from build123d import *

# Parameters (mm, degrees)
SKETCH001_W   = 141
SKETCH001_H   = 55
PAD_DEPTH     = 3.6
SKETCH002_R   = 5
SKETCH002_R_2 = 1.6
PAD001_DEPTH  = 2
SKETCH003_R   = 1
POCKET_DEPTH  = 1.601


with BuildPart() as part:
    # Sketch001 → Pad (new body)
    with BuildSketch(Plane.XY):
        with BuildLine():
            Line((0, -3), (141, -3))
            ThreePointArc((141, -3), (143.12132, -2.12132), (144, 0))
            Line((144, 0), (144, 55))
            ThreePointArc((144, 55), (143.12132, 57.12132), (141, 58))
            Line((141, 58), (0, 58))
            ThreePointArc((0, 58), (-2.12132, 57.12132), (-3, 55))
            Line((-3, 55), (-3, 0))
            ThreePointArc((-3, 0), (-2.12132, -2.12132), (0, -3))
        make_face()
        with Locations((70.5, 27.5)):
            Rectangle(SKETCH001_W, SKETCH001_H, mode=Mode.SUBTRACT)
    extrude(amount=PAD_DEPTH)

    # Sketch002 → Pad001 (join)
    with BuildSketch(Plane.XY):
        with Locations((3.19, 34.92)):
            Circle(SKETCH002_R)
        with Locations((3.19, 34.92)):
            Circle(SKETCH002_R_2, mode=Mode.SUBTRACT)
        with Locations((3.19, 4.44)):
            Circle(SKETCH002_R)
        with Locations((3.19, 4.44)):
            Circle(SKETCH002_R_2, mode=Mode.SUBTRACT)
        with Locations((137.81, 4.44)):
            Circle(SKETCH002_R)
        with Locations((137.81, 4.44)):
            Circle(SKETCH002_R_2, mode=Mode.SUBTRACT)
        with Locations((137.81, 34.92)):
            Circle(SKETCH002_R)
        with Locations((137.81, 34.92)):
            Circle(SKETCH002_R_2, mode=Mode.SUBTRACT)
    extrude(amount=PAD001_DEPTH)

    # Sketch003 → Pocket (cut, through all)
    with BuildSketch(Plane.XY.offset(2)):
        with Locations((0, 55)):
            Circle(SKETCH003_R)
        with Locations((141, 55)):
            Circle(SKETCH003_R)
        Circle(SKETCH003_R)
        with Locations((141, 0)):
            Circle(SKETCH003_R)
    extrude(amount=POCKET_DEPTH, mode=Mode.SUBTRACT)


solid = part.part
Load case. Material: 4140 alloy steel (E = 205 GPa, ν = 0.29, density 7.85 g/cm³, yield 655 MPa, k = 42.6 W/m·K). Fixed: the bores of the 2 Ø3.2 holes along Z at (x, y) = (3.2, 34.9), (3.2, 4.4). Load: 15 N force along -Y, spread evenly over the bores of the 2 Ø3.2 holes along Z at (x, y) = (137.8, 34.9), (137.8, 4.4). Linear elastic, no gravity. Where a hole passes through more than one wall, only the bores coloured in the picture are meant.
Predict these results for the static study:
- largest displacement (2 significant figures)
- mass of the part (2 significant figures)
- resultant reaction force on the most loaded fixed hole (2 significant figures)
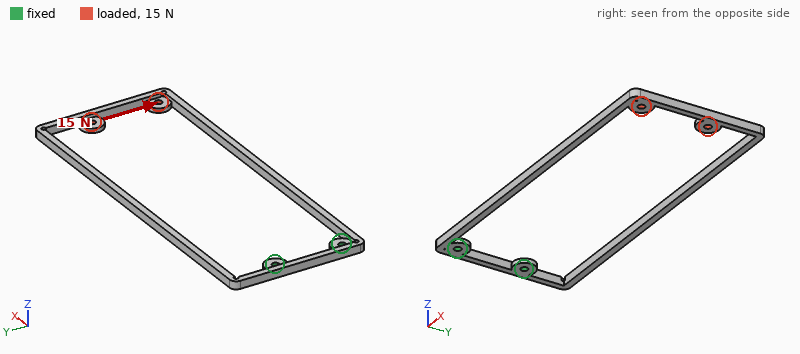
1.5 mm
38 g
24 N
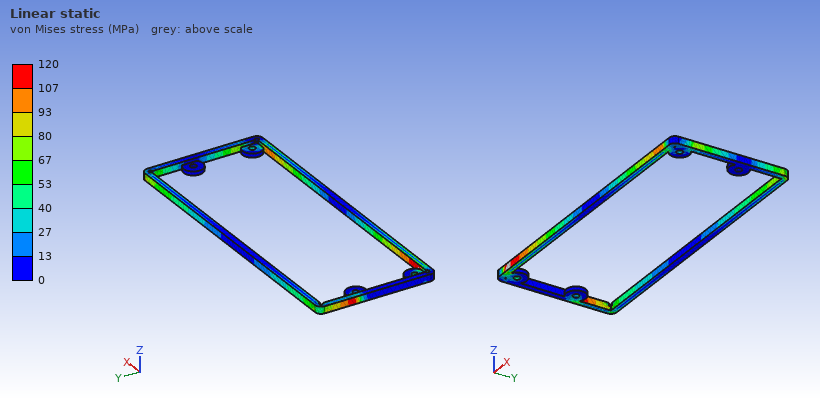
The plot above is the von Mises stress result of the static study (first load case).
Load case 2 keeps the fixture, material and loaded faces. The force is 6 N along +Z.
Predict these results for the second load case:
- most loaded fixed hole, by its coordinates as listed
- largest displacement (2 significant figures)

(3.2, 34.9)
1.6 mm
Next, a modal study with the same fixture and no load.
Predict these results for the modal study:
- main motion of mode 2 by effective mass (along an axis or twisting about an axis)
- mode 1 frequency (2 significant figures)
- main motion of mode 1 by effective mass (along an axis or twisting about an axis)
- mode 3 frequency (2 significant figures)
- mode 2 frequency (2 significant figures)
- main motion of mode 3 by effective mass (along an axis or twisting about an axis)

along Y
85 Hz
along Z
260 Hz
130 Hz
twisting about X
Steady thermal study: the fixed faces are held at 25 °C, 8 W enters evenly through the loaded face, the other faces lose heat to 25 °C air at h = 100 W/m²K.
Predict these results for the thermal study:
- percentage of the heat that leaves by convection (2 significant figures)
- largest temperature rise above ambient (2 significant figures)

100 %
83 K
